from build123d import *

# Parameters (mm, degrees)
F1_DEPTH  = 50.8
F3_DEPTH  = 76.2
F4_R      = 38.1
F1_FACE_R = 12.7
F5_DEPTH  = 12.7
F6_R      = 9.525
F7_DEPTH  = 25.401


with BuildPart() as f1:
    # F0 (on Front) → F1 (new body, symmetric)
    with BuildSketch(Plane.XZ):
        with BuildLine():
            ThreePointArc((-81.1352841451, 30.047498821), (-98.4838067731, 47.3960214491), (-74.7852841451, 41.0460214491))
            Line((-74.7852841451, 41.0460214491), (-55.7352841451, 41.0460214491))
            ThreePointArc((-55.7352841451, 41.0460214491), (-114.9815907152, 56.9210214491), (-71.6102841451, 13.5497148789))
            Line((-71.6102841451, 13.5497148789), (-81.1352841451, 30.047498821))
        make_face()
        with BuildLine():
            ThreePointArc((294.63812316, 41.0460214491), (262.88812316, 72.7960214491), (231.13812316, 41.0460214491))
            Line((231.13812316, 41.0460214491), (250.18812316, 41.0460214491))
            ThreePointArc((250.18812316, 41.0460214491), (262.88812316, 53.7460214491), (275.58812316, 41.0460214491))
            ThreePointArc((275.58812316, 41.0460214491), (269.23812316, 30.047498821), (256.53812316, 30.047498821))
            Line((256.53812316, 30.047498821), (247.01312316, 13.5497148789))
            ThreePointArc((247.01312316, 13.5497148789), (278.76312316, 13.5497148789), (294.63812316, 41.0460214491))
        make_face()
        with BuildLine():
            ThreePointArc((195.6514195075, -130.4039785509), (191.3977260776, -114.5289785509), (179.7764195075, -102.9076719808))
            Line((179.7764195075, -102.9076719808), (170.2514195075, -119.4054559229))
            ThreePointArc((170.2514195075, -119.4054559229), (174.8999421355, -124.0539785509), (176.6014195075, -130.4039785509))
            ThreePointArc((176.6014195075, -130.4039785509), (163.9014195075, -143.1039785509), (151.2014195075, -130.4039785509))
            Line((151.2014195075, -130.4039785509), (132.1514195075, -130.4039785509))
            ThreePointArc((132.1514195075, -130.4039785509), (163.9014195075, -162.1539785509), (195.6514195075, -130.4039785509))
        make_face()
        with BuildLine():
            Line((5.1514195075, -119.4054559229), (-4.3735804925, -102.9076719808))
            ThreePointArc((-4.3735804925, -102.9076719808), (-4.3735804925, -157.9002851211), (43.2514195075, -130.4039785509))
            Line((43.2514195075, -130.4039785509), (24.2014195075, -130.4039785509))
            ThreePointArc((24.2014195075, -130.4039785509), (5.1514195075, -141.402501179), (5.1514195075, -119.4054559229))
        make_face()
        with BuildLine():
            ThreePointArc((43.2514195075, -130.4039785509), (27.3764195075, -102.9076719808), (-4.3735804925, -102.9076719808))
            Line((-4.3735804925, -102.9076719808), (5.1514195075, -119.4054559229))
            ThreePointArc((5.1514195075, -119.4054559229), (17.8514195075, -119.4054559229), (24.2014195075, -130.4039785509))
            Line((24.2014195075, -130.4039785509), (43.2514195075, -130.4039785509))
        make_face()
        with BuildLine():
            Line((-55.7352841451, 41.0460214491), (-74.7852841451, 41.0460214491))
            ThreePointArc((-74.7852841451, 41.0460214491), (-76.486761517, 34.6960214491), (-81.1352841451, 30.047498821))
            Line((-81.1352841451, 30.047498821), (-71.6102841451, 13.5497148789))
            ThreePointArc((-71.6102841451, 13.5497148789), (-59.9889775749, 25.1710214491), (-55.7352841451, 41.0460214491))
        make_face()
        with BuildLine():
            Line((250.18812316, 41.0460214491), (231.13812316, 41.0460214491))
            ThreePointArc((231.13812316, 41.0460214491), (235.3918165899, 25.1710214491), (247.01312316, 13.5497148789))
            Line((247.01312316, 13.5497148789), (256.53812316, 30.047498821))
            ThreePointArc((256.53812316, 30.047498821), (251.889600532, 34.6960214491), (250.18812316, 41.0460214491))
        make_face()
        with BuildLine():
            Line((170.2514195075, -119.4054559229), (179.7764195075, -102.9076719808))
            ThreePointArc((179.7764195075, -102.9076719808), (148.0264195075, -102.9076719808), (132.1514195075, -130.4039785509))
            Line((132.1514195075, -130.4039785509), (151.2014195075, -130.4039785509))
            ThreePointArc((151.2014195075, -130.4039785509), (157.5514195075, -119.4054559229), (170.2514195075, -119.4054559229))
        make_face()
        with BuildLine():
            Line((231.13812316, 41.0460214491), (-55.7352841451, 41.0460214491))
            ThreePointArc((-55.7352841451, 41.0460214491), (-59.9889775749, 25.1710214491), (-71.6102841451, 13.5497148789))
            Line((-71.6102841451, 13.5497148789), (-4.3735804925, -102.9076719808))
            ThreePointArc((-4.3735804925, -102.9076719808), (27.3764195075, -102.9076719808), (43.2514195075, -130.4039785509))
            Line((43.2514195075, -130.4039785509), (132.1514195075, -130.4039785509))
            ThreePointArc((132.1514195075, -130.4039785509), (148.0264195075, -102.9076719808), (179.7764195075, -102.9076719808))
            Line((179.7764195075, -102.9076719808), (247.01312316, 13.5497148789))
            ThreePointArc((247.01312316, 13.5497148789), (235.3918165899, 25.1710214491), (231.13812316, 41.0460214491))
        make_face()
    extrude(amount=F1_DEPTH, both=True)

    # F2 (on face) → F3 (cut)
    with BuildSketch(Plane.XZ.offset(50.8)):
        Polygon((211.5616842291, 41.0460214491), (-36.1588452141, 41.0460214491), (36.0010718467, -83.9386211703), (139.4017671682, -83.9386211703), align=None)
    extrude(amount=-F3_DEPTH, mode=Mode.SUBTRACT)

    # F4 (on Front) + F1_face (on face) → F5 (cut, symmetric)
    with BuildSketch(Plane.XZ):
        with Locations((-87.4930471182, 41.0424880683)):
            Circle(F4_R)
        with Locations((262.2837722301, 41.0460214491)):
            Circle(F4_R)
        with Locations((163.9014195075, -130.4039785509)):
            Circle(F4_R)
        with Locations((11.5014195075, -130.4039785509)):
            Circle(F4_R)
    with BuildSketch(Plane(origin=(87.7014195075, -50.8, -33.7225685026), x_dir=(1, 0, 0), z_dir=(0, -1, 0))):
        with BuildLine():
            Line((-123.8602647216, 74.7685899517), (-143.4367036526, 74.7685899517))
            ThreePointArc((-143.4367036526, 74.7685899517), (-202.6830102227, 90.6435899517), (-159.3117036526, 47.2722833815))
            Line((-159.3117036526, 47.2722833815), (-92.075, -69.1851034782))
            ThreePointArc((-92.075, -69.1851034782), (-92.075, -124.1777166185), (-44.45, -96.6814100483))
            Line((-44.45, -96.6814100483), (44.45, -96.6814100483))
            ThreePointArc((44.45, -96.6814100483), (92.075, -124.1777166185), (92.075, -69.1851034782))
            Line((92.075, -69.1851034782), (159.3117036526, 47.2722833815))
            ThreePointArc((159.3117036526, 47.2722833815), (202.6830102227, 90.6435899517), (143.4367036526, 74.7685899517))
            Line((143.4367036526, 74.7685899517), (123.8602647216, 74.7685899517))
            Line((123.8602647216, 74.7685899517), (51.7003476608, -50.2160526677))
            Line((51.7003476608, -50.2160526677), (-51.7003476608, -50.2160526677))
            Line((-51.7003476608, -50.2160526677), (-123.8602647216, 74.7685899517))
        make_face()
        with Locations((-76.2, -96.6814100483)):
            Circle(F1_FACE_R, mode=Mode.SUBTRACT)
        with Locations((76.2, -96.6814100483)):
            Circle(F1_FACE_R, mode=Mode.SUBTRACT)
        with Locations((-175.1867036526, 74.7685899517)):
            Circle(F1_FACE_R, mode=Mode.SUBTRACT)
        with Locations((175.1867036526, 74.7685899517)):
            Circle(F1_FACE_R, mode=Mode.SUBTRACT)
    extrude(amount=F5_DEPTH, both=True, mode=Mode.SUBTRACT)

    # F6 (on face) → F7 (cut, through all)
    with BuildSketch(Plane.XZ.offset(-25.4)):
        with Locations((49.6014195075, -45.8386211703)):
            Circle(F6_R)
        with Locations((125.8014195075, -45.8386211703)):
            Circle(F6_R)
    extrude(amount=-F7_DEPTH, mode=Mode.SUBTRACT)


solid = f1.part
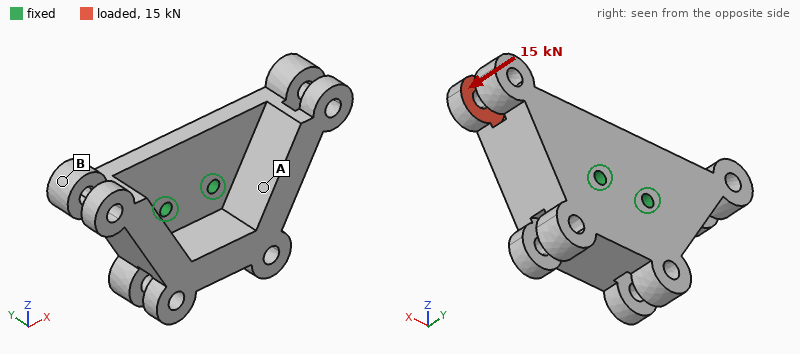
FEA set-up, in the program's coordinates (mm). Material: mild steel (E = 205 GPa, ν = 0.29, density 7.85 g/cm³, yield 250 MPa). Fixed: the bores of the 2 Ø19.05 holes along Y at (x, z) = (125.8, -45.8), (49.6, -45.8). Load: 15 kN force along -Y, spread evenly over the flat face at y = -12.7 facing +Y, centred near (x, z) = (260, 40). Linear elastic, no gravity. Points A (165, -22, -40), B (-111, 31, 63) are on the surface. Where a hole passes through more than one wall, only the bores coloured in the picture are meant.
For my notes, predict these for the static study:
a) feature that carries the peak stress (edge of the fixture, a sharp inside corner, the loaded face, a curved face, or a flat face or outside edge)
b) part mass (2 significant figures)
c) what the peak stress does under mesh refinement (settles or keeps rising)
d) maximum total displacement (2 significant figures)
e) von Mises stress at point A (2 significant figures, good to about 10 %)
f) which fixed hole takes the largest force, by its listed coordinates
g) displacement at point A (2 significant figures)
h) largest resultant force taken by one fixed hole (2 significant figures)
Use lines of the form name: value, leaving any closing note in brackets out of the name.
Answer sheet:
feature that carries the peak stress: edge of the fixture
part mass: 22 kg
what the peak stress does under mesh refinement: keeps rising
maximum total displacement: 0.33 mm
von Mises stress at point A: 26 MPa
which fixed hole takes the largest force, by its listed coordinates: (125.8, -45.8)
displacement at point A: 0.058 mm
largest resultant force taken by one fixed hole: 31 kN
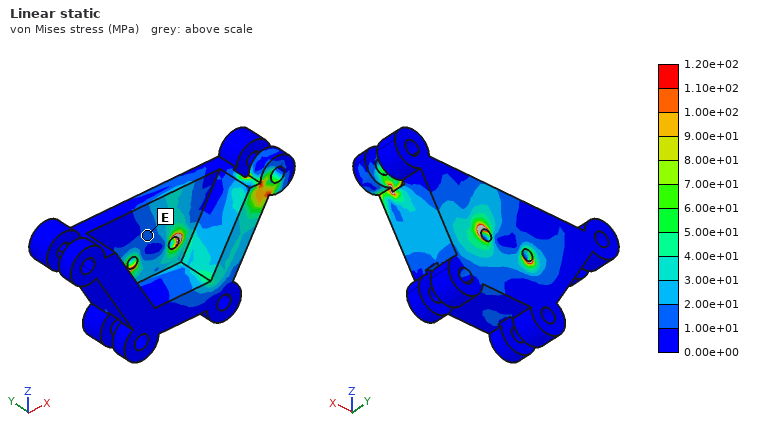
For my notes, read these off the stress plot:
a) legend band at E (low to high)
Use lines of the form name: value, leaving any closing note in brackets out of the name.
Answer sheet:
legend band at E: 1.00e+01 to 2.00e+01 MPa
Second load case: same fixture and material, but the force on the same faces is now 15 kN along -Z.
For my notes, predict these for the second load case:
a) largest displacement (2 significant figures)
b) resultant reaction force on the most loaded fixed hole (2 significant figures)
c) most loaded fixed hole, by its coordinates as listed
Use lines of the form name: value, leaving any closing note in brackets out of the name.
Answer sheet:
largest displacement: 0.17 mm
resultant reaction force on the most loaded fixed hole: 36 kN
most loaded fixed hole, by its coordinates as listed: (125.8, -45.8)
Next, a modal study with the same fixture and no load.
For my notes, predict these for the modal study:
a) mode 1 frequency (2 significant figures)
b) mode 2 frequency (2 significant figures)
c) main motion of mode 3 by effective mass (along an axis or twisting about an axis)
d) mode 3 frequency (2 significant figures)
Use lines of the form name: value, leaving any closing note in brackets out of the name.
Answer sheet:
mode 1 frequency: 760 Hz
mode 2 frequency: 910 Hz
main motion of mode 3 by effective mass: twisting about Y
mode 3 frequency: 1300 Hz
